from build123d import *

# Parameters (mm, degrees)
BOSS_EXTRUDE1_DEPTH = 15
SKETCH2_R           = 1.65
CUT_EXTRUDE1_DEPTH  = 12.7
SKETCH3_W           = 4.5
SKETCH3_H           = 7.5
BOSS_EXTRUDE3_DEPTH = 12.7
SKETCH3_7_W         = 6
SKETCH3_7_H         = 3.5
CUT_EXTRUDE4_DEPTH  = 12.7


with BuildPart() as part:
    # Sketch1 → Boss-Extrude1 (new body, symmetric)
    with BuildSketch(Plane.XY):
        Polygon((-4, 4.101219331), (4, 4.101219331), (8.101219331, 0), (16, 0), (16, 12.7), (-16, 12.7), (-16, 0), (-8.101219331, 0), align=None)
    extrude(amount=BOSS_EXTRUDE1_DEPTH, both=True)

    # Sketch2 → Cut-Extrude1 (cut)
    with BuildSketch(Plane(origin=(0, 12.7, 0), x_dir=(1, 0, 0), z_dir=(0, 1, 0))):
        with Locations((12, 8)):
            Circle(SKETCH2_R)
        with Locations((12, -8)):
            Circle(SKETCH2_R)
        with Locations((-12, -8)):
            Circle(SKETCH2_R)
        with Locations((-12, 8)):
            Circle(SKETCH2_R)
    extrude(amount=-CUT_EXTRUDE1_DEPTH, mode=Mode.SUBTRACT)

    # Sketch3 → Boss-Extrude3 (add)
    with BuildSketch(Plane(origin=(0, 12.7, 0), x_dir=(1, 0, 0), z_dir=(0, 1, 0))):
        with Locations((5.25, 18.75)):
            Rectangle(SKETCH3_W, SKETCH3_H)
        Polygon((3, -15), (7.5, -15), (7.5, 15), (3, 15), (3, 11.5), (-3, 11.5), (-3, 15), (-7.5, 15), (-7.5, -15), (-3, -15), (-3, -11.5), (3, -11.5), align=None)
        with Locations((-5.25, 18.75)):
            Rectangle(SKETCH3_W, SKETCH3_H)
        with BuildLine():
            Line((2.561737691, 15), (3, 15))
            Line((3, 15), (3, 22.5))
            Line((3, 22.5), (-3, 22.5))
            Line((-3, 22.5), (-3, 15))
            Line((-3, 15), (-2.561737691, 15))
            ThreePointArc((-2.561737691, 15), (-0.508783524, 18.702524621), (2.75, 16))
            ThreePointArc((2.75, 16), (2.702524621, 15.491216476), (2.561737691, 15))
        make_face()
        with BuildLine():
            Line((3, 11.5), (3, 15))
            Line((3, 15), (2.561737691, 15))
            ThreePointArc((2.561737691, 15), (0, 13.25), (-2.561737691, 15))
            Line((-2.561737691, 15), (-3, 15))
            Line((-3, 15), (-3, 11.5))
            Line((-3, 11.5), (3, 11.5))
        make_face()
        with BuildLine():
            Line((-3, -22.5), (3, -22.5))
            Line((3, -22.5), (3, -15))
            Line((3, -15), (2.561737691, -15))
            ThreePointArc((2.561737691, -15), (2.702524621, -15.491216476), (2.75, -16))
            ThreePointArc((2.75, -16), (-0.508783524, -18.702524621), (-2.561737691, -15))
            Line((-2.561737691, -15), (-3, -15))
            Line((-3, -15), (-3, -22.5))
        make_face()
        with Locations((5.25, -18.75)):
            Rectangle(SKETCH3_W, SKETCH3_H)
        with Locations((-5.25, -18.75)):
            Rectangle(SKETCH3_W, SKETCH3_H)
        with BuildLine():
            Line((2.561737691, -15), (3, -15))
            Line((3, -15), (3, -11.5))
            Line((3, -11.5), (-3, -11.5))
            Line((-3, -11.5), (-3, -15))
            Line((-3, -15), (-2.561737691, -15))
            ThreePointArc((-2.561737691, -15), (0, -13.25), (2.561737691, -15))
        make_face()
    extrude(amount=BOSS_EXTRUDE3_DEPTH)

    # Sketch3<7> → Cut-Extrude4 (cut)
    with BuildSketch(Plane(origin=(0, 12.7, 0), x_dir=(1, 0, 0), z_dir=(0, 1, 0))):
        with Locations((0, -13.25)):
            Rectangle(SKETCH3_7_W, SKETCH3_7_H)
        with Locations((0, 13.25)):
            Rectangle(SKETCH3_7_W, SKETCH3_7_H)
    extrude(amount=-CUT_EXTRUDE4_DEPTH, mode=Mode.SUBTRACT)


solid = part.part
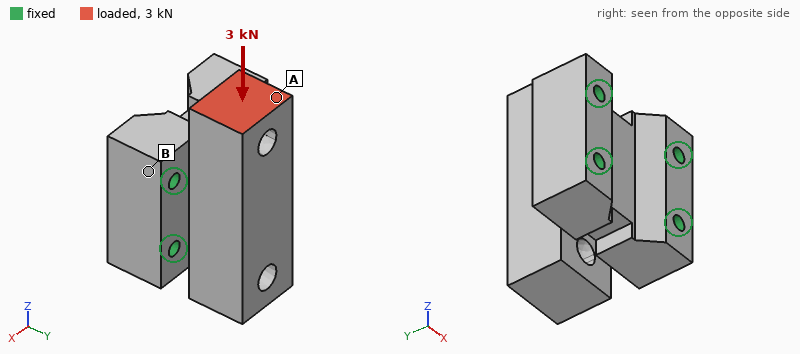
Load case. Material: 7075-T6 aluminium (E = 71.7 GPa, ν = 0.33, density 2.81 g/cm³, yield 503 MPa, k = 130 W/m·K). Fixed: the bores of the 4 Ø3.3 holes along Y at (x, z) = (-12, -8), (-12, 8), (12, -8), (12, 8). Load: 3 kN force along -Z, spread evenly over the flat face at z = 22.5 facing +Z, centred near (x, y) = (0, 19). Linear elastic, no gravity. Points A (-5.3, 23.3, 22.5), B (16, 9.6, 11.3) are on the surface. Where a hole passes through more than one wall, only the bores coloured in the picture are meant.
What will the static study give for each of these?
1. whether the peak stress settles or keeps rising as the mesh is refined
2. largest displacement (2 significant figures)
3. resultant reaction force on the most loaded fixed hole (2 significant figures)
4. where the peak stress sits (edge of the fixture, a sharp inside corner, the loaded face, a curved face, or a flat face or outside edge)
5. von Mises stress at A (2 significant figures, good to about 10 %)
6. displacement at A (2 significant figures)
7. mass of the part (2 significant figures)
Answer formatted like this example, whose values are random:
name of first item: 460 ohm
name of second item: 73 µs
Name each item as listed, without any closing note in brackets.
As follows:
whether the peak stress settles or keeps rising as the mesh is refined: keeps rising
largest displacement: 19 µm
resultant reaction force on the most loaded fixed hole: 1.2 kN
where the peak stress sits: edge of the fixture
von Mises stress at A: 16 MPa
displacement at A: 17 µm
mass of the part: 50 g
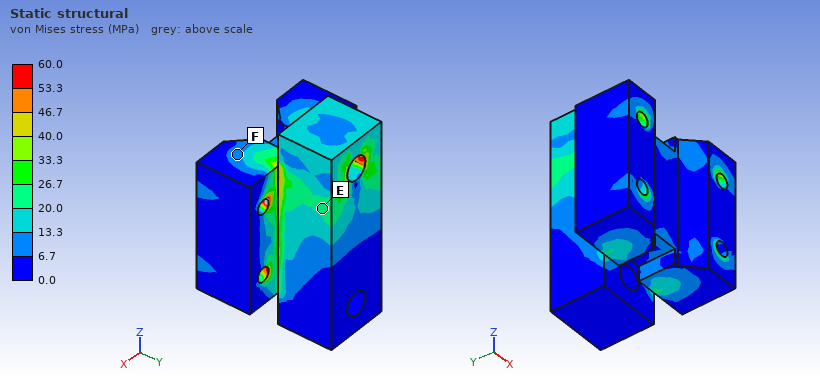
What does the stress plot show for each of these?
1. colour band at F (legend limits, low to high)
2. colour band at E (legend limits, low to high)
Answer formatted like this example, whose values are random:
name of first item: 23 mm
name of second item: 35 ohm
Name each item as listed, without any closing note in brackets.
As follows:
colour band at F: 6.7 to 13.3 MPa
colour band at E: 20.0 to 26.7 MPa
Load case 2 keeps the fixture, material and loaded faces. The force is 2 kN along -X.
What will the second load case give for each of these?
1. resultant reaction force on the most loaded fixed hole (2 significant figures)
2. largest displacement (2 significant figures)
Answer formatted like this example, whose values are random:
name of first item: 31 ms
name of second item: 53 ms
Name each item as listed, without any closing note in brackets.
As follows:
resultant reaction force on the most loaded fixed hole: 1.5 kN
largest displacement: 31 µm
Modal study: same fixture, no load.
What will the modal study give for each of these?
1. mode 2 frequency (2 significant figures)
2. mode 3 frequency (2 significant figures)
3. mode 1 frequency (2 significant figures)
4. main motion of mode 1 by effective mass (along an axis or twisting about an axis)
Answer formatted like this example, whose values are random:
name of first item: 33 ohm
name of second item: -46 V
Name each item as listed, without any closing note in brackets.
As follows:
mode 2 frequency: 24 kHz
mode 3 frequency: 24 kHz
mode 1 frequency: 18 kHz
main motion of mode 1 by effective mass: along Z
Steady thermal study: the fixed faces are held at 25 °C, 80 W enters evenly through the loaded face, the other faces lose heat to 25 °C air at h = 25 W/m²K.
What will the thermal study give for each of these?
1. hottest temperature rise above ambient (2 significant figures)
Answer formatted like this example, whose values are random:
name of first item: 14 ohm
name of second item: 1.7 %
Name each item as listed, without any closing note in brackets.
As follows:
hottest temperature rise above ambient: 75 K
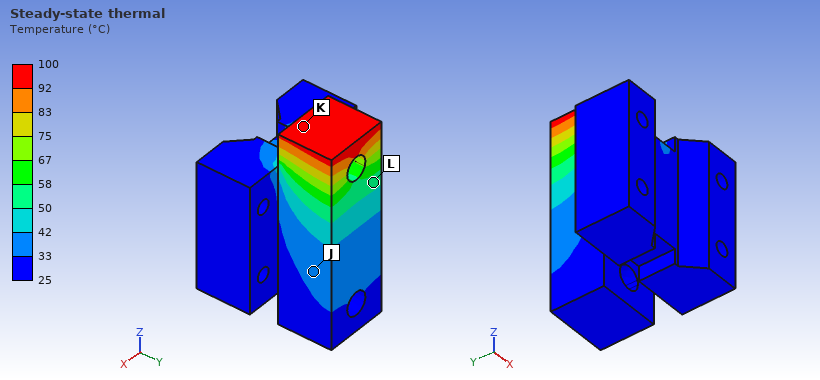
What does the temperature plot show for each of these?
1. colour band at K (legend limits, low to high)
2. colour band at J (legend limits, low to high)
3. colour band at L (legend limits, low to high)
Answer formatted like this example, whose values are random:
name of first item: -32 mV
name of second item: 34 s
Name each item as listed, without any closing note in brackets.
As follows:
colour band at K: 92 to 100 °C
colour band at J: 33 to 42 °C
colour band at L: 50 to 58 °C
